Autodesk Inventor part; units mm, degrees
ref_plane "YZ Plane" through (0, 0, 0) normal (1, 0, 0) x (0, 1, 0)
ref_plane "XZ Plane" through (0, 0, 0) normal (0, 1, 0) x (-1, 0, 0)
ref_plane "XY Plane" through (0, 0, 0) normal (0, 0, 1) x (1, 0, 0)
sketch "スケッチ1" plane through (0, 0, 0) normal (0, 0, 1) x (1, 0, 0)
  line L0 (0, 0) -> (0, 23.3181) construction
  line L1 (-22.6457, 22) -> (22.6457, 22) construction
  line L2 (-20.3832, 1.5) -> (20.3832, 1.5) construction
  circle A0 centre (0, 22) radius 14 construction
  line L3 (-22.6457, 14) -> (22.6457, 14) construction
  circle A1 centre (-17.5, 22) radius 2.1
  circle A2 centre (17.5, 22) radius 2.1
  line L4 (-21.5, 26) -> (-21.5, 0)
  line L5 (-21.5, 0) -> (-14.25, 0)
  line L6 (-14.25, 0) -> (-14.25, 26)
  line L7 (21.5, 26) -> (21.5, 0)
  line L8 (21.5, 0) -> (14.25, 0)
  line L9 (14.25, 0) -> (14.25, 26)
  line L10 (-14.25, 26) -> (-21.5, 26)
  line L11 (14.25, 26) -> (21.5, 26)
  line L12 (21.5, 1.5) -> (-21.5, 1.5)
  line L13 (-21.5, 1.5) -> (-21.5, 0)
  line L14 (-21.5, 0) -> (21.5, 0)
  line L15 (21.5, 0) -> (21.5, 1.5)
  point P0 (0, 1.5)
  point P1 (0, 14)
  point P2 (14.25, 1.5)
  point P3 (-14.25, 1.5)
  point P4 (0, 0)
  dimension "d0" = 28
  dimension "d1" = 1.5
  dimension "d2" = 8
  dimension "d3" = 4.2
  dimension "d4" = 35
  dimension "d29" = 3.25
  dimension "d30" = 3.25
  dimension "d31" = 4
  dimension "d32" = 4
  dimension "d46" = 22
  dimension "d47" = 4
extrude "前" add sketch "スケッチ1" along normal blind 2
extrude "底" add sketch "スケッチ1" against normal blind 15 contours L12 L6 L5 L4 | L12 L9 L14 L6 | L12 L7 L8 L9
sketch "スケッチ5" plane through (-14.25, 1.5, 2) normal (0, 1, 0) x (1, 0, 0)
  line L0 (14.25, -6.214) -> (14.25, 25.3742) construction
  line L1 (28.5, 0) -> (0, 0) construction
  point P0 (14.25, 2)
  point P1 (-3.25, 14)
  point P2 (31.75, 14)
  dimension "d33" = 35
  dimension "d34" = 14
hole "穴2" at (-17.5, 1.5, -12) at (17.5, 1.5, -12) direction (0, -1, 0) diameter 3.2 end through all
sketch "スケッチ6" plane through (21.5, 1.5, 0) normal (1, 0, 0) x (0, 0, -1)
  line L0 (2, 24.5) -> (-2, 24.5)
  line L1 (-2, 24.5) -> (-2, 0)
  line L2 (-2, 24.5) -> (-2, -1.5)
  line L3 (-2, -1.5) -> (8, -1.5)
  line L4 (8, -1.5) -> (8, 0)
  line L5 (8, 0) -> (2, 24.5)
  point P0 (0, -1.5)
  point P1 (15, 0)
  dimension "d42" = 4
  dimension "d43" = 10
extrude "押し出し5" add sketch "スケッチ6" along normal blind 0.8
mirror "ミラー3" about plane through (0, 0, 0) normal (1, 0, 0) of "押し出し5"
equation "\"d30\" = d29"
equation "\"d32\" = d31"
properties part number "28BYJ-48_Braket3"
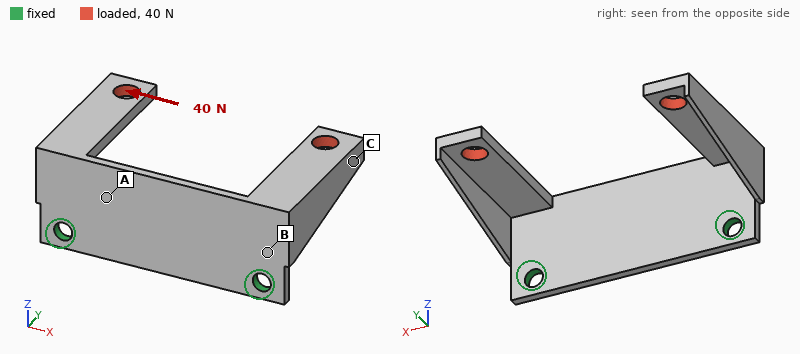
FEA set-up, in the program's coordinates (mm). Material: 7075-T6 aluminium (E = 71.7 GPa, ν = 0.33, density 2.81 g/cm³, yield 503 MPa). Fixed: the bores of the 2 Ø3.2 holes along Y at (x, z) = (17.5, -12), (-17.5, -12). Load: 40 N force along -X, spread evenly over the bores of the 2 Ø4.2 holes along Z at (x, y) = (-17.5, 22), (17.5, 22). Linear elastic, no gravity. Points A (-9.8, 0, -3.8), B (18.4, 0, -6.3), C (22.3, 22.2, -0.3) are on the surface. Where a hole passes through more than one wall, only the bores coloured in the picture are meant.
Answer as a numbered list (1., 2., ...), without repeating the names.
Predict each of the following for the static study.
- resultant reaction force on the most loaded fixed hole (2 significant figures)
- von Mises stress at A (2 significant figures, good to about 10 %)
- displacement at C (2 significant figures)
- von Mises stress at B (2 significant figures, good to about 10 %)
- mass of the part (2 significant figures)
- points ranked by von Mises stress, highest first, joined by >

1. 27 N
2. 23 MPa
3. 0.21 mm
4. 52 MPa
5. 5.7 g
6. B > A > C
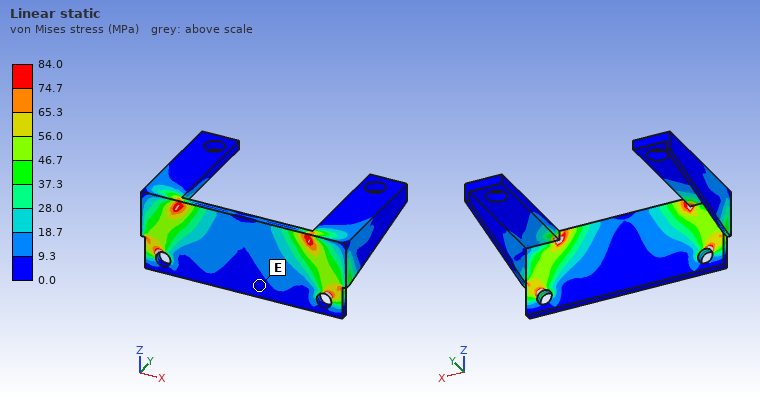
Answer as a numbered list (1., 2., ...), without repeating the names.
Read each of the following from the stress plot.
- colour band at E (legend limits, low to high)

1. 0.0 to 9.3 MPa
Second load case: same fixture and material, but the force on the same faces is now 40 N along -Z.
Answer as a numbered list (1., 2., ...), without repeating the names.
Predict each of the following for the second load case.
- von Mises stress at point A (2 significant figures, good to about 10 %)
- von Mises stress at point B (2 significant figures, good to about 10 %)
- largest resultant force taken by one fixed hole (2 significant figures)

1. 27 MPa
2. 71 MPa
3. 20 N
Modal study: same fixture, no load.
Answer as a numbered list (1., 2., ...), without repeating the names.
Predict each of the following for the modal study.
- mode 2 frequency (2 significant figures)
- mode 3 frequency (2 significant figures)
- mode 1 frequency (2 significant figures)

1. 1600 Hz
2. 2100 Hz
3. 1500 Hz
